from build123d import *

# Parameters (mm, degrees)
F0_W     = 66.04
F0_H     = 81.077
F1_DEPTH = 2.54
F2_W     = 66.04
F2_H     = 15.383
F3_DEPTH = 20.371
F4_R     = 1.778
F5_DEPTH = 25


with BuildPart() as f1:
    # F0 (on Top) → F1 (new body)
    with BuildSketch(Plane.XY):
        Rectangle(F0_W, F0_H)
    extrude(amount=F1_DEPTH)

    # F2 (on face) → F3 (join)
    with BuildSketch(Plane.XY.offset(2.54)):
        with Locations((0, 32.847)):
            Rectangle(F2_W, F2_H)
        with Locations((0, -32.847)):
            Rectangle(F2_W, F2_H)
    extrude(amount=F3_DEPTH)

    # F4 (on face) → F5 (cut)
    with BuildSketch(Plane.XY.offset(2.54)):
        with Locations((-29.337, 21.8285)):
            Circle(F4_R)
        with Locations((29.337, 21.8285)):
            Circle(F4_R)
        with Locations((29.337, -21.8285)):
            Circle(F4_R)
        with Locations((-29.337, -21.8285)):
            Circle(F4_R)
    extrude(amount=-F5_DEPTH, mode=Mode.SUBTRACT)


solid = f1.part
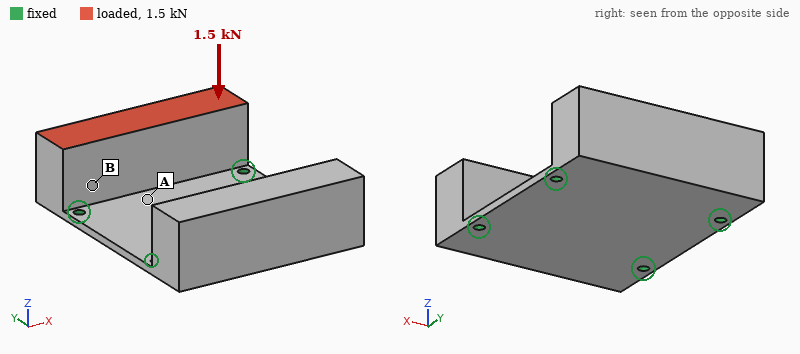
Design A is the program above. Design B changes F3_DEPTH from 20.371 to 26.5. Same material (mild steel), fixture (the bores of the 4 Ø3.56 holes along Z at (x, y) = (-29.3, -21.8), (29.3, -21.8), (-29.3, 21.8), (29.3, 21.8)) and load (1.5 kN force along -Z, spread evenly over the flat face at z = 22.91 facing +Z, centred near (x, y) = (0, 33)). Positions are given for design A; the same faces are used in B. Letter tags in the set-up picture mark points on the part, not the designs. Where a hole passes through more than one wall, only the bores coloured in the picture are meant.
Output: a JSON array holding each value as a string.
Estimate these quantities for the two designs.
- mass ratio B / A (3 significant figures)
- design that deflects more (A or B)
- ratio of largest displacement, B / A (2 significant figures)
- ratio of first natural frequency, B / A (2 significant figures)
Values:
["1.23", "B", "1.2", "0.75"]
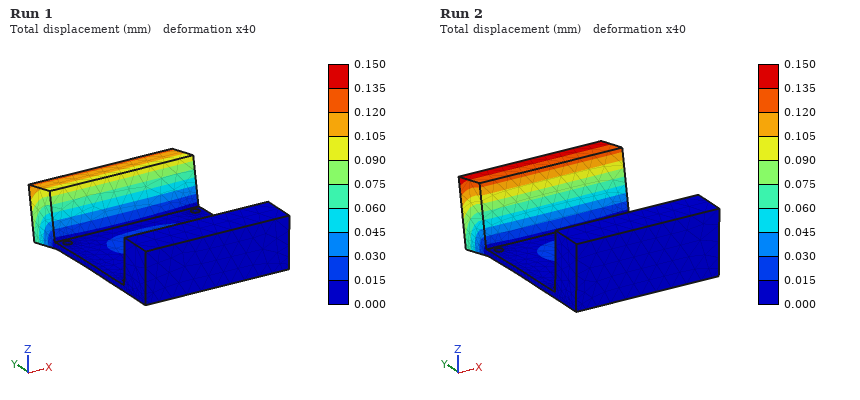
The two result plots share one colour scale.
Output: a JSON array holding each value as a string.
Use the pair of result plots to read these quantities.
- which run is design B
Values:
["Run 2"]
